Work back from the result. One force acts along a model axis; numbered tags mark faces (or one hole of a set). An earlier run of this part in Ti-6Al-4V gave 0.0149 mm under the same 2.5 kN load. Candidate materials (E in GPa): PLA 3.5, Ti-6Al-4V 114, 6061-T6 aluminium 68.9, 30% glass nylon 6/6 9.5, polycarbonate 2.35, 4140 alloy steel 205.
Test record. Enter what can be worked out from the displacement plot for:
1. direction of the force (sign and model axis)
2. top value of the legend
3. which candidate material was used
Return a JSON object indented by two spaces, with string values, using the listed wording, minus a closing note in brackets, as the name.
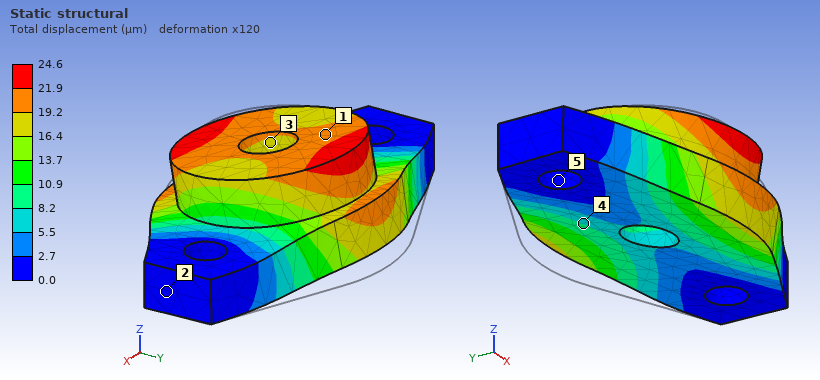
{
  "direction of the force": "-Y",
  "top value of the legend": "24.6 µm",
  "which candidate material was used": "6061-T6 aluminium"
}
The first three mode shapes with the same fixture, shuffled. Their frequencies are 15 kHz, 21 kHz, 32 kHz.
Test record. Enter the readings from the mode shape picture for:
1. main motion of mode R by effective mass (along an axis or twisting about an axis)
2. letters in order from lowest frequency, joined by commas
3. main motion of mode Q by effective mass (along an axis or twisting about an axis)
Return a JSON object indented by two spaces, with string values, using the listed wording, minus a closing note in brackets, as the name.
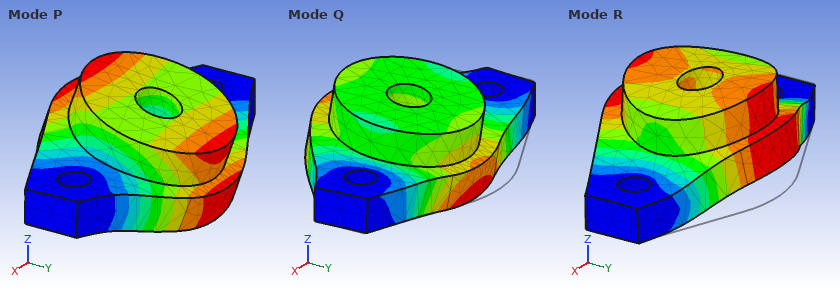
{
  "main motion of mode R by effective mass": "along Z",
  "letters in order from lowest frequency, joined by commas": "P, R, Q",
  "main motion of mode Q by effective mass": "along Y"
}
